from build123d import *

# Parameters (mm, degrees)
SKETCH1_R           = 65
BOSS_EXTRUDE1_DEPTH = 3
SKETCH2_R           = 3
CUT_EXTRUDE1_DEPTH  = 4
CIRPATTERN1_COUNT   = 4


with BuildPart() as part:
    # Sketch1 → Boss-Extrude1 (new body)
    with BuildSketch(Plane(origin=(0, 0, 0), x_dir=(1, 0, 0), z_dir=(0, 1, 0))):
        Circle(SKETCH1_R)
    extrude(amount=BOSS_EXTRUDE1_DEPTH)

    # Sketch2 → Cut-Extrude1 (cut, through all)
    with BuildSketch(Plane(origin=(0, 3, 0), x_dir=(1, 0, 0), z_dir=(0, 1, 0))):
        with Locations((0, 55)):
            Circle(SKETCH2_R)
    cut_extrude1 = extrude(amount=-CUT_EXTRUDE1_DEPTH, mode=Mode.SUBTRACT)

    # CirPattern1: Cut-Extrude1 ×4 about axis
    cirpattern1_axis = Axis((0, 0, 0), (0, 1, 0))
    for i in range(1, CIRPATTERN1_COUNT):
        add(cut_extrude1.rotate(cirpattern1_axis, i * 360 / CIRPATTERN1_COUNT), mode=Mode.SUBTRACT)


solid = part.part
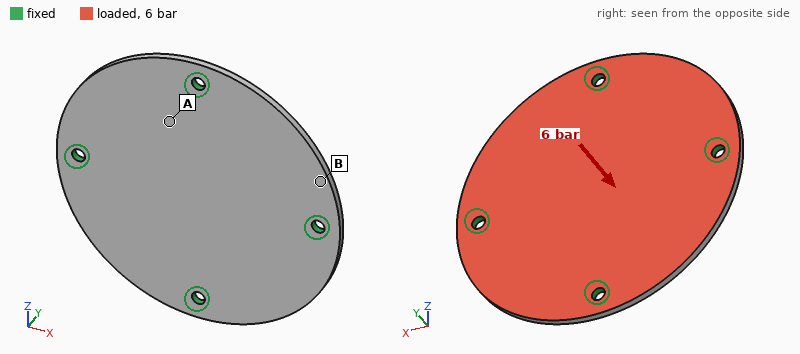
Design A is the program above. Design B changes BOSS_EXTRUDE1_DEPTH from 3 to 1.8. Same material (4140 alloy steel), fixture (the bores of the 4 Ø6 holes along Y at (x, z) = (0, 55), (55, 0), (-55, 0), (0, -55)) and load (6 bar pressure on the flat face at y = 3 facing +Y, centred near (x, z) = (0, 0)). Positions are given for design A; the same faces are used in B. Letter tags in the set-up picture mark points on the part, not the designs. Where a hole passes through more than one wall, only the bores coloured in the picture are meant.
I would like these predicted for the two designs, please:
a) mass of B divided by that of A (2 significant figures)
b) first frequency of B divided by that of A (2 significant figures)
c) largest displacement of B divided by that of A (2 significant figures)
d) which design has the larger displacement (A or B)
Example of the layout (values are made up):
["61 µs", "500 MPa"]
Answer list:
["0.60", "0.61", "4.5", "B"]
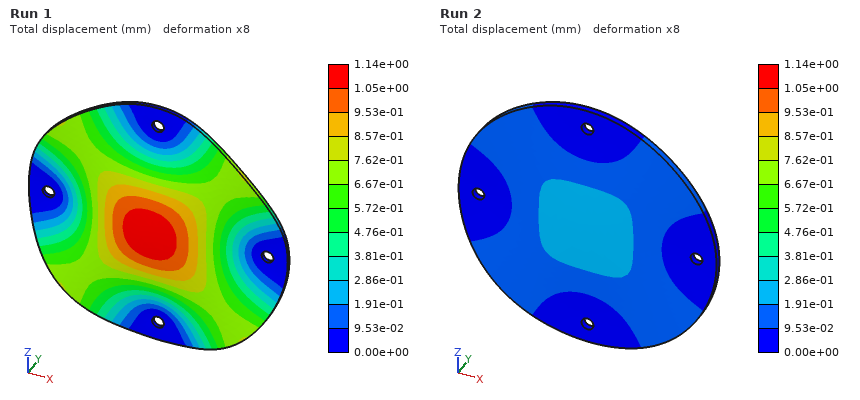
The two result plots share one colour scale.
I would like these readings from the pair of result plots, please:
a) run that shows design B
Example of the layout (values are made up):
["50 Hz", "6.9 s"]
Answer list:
["Run 1"]
